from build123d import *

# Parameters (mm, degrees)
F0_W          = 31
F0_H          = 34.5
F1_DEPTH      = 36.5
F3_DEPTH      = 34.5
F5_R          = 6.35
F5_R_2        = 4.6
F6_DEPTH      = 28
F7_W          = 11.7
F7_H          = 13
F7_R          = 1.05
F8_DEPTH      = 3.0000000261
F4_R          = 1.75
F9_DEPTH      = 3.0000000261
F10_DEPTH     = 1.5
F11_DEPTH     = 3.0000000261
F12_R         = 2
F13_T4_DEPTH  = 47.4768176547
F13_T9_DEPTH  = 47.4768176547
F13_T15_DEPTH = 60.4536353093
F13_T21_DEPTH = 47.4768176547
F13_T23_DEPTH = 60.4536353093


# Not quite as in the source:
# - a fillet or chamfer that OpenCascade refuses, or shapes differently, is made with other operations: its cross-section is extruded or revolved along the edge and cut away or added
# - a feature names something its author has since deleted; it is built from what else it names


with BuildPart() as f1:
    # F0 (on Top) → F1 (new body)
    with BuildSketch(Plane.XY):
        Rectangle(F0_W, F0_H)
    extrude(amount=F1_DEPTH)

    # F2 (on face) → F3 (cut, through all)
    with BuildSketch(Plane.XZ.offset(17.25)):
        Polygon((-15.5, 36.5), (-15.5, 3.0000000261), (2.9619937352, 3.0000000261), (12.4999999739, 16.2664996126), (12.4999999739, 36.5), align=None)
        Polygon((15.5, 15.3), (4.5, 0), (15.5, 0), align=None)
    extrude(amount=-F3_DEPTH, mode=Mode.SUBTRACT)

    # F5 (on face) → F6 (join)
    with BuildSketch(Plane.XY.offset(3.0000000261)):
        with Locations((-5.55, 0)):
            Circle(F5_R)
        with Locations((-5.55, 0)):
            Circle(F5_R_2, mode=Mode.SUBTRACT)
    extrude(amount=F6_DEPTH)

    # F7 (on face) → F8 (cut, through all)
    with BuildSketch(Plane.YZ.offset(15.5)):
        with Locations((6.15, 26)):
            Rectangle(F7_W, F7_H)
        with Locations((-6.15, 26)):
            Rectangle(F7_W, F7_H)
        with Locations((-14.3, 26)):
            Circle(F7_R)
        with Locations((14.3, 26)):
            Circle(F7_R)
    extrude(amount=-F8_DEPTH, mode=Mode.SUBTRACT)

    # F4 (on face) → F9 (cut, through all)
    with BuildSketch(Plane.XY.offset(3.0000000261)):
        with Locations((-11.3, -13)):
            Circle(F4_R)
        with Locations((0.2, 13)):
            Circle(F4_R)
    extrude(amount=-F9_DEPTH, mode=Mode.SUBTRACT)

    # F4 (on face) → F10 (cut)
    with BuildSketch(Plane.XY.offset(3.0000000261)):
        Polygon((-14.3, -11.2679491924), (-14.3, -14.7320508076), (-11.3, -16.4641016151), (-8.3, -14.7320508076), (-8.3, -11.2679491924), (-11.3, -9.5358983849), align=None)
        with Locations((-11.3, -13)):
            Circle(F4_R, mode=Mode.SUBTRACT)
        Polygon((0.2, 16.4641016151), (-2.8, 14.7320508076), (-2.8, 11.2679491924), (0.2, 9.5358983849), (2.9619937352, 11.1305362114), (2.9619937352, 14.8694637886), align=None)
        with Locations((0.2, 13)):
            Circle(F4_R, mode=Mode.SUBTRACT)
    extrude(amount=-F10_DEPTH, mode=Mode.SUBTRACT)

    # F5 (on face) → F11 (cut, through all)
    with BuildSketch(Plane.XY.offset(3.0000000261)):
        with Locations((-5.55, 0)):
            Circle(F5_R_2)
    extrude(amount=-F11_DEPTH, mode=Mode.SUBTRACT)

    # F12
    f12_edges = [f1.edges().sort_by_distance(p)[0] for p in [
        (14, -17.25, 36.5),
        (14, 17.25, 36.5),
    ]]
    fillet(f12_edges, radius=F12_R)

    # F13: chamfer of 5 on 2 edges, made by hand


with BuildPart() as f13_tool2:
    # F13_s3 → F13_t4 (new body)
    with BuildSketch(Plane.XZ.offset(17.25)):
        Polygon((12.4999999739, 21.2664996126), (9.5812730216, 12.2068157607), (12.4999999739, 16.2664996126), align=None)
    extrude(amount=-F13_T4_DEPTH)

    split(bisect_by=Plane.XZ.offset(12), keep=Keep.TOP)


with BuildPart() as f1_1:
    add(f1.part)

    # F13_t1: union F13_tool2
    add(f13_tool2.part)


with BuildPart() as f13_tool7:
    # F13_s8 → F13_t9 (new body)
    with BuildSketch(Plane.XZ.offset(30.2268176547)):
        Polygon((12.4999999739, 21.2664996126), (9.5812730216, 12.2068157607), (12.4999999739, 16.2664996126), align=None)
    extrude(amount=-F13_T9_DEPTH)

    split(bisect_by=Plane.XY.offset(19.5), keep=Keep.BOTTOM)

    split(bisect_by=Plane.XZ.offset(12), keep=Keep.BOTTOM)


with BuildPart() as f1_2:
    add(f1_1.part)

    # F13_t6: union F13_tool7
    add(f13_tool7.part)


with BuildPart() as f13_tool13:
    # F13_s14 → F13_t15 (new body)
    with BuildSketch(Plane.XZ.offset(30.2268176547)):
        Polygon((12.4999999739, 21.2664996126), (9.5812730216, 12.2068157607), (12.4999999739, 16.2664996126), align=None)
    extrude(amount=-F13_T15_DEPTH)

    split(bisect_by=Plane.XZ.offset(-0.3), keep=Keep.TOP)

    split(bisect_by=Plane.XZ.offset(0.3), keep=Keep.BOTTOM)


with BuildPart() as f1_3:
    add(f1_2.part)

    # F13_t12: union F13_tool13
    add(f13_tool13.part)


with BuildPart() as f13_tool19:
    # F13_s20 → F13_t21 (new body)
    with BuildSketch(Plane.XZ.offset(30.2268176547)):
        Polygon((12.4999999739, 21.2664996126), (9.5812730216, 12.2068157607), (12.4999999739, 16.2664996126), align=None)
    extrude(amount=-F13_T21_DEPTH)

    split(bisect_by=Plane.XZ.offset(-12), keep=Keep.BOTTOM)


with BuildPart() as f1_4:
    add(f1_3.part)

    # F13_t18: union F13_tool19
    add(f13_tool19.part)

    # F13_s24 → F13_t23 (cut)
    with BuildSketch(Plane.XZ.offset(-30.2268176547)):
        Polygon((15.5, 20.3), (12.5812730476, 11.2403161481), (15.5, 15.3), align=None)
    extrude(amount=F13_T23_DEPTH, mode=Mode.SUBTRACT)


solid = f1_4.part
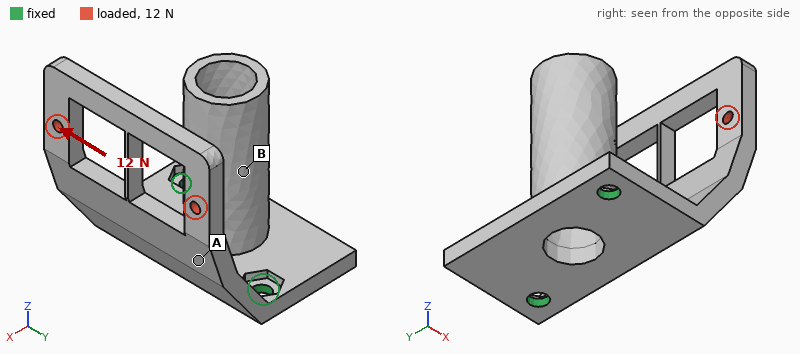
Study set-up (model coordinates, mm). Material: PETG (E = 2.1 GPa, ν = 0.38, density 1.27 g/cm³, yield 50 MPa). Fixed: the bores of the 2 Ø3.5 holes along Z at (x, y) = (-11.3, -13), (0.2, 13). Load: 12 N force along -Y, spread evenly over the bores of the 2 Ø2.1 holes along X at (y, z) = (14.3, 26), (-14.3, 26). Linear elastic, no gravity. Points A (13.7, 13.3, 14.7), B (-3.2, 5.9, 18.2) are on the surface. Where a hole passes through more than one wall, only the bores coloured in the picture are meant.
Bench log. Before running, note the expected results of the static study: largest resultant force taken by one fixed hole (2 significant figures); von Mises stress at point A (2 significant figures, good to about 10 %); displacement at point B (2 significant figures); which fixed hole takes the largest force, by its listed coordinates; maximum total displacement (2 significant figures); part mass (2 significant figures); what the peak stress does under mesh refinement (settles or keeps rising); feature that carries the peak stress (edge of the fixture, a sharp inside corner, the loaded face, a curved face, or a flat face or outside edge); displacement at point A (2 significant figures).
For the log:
15 N
1.2 MPa
0.13 mm
(-11.3, -13)
0.58 mm
8.1 g
keeps rising
edge of the fixture
0.10 mm
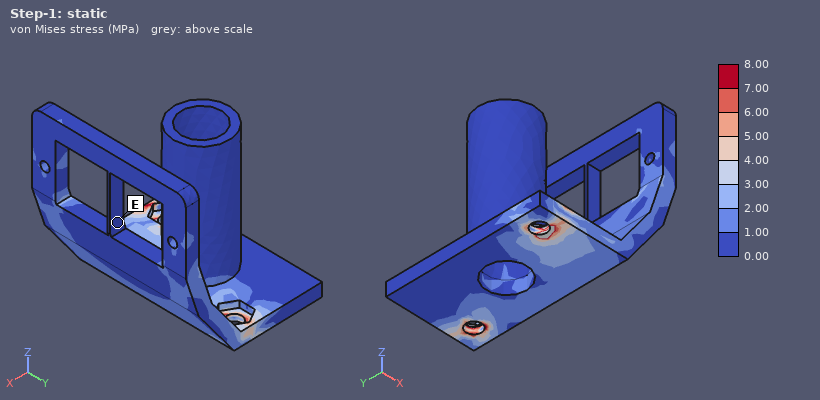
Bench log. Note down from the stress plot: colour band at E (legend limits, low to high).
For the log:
0.00 to 1.00 MPa
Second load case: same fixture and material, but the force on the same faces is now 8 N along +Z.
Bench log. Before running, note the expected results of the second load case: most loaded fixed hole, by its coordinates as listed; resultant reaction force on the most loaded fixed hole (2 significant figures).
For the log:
(0.2, 13)
6.5 N
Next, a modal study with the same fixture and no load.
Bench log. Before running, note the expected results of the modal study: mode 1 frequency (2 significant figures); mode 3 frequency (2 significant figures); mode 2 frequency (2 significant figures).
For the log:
320 Hz
920 Hz
650 Hz
